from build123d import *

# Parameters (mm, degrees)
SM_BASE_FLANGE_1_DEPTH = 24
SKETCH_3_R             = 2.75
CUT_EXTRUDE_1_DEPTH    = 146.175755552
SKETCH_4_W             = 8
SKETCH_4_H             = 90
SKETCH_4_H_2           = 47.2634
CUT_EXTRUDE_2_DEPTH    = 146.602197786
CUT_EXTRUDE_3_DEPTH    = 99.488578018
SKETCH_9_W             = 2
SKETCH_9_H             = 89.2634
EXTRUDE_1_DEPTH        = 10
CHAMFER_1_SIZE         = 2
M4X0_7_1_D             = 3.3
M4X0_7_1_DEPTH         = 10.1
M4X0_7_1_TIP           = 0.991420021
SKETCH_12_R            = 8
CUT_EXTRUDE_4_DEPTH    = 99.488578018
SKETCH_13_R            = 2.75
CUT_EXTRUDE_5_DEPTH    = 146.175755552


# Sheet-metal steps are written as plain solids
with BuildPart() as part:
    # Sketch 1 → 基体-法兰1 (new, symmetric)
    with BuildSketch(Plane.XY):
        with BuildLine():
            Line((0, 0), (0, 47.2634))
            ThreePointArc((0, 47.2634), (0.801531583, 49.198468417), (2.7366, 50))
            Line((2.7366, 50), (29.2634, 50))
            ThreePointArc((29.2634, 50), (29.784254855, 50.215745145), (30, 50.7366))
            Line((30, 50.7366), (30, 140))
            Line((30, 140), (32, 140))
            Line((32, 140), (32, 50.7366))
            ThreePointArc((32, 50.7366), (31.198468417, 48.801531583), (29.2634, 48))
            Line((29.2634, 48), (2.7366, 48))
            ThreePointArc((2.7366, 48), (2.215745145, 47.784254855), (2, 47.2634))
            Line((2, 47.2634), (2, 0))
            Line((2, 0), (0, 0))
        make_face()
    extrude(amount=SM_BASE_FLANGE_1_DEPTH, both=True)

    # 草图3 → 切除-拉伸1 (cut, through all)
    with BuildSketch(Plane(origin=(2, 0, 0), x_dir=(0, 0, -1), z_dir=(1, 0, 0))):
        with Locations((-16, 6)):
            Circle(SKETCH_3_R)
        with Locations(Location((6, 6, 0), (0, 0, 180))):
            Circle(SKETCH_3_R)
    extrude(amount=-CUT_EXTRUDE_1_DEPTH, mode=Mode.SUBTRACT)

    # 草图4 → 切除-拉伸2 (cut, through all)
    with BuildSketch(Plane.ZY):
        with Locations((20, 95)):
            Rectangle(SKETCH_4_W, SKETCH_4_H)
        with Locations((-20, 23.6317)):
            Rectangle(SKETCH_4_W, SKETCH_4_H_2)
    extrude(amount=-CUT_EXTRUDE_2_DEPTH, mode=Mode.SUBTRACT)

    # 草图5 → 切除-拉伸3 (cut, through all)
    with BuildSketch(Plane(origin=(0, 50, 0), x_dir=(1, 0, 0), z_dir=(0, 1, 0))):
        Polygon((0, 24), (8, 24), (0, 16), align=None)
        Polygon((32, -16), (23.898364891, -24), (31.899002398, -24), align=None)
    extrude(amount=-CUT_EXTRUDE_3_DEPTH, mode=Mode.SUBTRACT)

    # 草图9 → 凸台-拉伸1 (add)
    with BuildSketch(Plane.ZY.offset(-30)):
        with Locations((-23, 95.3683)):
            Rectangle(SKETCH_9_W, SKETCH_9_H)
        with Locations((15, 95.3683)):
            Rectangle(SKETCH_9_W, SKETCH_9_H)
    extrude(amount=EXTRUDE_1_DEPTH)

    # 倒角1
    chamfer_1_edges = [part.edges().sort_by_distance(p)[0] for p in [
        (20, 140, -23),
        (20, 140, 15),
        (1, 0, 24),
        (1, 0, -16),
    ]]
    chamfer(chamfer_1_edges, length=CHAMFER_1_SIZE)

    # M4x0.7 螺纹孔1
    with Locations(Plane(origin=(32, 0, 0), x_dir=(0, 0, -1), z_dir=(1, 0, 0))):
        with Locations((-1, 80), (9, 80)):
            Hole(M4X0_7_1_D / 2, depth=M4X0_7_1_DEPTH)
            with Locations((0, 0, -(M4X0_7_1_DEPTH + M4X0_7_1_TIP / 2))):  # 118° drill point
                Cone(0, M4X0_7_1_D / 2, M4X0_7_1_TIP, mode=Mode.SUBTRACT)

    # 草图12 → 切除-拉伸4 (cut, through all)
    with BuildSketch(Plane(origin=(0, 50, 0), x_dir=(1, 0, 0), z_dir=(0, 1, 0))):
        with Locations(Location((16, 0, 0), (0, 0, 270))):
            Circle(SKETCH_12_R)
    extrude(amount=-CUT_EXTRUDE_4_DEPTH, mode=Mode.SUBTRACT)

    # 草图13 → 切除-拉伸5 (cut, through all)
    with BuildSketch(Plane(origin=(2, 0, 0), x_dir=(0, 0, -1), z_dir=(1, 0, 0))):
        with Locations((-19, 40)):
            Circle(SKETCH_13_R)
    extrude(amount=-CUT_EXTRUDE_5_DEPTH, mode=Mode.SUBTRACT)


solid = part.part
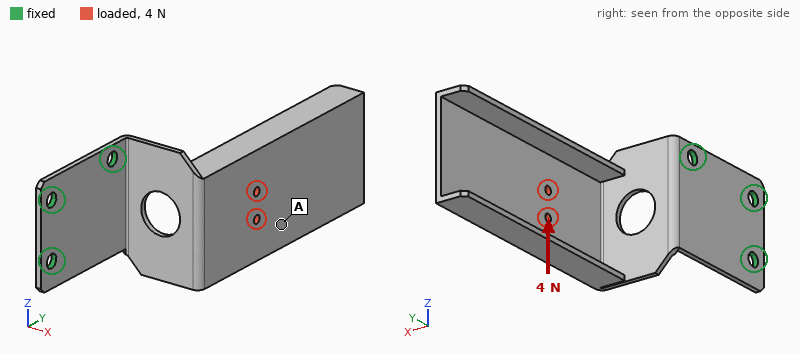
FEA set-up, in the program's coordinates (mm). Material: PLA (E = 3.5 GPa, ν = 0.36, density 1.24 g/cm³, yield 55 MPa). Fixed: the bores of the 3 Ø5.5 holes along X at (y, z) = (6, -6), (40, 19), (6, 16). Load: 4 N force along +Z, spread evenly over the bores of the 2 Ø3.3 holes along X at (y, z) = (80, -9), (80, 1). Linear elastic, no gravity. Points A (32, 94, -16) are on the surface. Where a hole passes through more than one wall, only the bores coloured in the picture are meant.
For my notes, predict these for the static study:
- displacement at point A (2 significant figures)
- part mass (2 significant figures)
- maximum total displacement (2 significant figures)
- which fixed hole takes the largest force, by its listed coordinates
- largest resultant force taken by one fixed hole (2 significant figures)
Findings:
0.90 mm
21 g
1.6 mm
(40, 19)
7.0 N
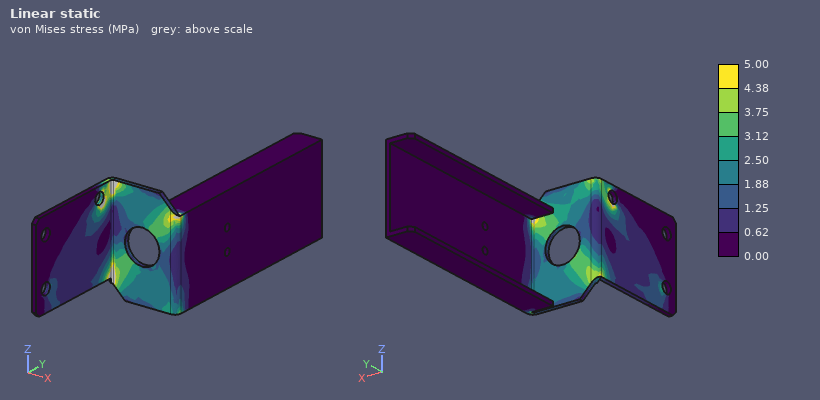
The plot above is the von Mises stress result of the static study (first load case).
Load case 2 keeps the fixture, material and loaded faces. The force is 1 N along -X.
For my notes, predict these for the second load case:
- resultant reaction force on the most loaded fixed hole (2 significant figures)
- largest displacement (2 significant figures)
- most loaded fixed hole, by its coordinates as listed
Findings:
1.5 N
1.7 mm
(40, 19)
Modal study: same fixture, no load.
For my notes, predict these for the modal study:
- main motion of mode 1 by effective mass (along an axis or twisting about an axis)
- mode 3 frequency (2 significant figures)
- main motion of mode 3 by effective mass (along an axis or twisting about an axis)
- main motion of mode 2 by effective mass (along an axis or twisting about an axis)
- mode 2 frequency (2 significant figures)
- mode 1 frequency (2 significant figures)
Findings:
along X
170 Hz
along Y
along Z
67 Hz
33 Hz
